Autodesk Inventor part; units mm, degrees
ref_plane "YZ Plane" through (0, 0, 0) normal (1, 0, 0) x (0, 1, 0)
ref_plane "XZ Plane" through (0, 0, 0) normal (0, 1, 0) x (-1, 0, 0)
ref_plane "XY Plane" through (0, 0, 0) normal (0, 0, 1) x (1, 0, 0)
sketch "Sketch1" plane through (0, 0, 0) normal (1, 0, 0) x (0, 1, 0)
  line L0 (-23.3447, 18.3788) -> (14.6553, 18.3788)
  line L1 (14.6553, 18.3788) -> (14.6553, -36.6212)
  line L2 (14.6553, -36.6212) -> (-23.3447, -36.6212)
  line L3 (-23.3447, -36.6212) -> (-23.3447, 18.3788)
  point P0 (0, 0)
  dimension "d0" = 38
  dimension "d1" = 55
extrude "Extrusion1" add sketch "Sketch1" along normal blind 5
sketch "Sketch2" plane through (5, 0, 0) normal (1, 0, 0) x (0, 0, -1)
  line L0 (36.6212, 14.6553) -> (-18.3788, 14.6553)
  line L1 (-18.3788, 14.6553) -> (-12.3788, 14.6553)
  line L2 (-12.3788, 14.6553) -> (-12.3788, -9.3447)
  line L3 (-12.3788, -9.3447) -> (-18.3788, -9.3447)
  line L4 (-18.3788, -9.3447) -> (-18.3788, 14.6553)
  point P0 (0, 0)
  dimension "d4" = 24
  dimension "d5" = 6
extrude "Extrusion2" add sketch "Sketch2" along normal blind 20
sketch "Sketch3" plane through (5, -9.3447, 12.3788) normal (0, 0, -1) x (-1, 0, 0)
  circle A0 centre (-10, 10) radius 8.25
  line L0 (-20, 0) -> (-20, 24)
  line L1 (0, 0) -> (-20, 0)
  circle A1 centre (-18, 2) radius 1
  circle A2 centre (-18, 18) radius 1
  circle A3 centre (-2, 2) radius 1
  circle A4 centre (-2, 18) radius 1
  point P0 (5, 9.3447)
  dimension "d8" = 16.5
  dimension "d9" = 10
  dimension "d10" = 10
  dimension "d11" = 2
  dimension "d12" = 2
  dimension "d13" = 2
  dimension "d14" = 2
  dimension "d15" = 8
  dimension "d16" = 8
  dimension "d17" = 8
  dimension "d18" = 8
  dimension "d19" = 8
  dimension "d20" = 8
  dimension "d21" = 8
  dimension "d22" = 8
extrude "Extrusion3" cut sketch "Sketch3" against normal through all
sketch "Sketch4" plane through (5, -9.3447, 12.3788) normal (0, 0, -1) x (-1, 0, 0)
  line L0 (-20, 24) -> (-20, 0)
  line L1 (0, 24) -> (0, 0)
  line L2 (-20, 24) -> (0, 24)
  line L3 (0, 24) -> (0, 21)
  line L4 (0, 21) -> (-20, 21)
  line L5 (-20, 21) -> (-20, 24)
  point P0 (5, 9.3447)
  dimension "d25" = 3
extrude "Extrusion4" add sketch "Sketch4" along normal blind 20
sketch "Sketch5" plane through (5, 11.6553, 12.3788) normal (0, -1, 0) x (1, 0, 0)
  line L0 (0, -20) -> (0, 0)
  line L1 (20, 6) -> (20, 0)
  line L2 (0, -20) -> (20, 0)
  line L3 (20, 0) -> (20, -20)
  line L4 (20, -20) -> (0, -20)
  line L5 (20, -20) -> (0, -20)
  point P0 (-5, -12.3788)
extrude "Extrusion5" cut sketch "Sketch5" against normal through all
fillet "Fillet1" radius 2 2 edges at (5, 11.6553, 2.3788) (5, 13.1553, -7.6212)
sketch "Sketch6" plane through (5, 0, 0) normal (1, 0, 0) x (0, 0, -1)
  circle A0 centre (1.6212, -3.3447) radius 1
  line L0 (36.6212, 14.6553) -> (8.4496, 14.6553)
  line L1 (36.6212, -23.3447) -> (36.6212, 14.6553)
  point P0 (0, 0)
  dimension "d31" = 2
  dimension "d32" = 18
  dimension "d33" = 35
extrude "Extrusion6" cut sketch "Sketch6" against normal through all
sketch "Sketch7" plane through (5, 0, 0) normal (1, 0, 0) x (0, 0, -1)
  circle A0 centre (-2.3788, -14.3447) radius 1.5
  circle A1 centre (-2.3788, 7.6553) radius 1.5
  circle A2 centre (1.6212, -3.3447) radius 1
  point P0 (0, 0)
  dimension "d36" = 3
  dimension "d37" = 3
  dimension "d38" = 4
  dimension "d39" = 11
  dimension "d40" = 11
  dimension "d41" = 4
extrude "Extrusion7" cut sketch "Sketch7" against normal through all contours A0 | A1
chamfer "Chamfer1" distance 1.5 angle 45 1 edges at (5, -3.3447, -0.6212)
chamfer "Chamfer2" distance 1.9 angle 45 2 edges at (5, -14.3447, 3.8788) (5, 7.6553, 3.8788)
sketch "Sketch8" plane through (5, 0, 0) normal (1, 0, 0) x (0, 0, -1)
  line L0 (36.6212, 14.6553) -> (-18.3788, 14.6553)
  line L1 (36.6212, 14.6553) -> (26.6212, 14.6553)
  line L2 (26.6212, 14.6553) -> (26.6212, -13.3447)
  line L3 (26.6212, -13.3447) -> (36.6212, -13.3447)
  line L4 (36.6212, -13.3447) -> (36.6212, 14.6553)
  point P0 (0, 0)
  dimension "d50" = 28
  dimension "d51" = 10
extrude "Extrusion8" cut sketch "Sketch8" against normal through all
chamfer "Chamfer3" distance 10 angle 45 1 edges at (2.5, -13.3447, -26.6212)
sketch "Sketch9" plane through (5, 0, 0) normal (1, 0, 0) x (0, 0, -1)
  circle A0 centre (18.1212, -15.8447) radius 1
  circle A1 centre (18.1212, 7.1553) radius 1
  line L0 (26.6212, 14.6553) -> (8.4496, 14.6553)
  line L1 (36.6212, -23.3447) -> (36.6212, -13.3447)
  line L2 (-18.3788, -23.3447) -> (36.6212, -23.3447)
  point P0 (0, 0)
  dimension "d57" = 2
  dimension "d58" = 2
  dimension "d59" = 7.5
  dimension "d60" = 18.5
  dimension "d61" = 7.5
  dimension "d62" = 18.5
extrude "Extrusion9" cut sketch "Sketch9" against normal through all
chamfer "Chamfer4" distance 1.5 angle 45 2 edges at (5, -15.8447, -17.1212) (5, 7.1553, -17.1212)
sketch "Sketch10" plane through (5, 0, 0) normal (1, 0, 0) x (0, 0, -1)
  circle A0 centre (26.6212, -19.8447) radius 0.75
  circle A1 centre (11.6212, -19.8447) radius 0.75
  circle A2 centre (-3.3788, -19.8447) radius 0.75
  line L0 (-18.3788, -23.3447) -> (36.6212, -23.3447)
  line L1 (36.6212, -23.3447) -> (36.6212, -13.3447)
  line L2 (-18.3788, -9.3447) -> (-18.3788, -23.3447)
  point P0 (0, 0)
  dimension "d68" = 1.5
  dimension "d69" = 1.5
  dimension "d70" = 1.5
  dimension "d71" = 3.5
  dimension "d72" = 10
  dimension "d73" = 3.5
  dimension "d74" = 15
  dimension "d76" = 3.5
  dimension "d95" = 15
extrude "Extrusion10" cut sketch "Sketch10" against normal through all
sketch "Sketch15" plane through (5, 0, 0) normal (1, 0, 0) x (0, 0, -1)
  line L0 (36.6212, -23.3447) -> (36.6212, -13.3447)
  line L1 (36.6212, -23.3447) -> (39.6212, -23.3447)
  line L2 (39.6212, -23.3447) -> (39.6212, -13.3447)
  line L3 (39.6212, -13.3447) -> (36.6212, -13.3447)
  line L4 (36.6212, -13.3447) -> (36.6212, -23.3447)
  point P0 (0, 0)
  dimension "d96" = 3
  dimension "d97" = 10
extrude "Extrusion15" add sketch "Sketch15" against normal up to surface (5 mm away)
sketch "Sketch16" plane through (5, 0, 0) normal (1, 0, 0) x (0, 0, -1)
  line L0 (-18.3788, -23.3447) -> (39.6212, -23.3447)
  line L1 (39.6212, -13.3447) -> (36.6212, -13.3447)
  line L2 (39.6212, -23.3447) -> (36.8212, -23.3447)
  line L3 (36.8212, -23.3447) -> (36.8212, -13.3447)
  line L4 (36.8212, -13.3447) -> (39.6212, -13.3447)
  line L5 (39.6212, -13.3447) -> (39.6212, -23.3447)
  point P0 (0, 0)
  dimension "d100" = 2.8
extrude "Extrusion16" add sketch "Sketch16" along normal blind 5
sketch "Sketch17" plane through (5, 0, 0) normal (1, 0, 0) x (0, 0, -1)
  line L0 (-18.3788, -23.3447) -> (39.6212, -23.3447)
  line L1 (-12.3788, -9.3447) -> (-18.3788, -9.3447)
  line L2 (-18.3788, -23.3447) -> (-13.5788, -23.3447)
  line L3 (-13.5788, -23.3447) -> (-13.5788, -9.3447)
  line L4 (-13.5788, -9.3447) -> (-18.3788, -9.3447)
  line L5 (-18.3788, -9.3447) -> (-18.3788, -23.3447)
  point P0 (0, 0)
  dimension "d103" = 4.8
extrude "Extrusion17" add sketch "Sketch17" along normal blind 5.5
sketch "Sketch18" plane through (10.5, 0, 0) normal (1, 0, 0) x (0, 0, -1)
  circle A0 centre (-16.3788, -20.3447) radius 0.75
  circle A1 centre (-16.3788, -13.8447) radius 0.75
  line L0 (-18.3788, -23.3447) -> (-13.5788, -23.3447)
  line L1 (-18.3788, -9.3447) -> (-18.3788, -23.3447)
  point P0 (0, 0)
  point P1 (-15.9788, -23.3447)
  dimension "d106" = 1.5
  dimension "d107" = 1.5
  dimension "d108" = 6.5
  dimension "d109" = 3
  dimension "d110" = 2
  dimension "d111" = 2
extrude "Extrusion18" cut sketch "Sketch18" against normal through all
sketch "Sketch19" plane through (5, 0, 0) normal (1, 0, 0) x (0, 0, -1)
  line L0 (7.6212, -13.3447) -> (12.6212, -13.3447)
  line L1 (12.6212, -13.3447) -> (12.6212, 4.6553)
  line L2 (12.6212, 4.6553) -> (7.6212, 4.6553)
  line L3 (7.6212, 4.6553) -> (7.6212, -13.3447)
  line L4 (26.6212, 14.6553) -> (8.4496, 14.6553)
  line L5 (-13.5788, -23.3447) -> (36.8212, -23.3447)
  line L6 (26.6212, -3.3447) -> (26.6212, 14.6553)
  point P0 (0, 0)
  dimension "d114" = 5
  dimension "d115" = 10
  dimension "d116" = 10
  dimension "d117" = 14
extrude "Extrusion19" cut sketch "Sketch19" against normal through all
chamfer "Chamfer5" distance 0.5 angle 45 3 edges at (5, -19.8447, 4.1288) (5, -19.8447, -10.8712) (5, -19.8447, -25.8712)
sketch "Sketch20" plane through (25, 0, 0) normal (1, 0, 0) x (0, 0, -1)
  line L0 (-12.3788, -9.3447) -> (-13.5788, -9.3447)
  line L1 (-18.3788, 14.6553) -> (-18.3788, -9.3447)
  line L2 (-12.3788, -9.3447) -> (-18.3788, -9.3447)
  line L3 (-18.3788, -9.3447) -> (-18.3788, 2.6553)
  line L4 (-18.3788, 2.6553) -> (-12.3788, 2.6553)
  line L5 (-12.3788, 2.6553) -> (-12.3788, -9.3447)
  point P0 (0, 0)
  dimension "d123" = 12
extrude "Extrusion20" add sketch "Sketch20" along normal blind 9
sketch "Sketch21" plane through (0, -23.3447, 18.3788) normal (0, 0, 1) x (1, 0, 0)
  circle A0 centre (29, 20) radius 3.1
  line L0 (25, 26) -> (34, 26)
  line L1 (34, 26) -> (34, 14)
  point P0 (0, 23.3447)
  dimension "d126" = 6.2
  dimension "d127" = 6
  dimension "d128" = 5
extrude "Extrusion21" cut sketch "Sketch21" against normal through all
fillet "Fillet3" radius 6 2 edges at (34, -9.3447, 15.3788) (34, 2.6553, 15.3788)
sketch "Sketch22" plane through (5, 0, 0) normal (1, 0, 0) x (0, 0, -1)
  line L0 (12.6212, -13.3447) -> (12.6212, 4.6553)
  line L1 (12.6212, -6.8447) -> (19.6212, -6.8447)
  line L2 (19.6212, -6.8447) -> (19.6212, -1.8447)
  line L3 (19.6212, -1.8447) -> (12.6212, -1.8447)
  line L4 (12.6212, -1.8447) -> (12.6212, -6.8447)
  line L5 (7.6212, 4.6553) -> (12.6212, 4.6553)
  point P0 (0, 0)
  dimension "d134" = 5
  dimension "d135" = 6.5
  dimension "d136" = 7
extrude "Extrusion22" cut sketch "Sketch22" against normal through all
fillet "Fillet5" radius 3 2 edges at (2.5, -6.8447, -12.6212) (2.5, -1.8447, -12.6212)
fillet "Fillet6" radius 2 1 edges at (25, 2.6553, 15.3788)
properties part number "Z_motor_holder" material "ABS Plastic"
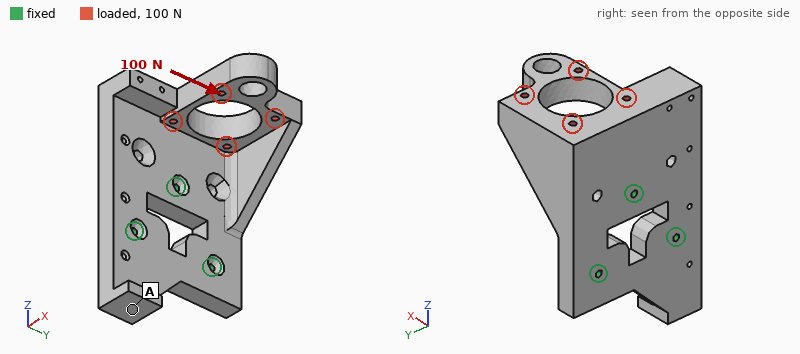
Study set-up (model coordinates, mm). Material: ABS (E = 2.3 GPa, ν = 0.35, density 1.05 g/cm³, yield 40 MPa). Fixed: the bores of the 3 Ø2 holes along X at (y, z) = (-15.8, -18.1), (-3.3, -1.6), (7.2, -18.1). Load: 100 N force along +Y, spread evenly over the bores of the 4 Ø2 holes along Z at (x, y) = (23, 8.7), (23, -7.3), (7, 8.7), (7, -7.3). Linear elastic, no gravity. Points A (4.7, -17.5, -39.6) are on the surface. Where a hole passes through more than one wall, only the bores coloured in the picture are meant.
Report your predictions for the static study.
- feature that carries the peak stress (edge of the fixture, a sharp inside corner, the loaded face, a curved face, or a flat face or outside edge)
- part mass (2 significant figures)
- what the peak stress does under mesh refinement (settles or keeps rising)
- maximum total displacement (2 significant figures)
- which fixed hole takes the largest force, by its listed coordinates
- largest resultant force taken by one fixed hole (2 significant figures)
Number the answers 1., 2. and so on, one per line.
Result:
1. edge of the fixture
2. 12 g
3. keeps rising
4. 0.83 mm
5. (-3.3, -1.6)
6. 110 N
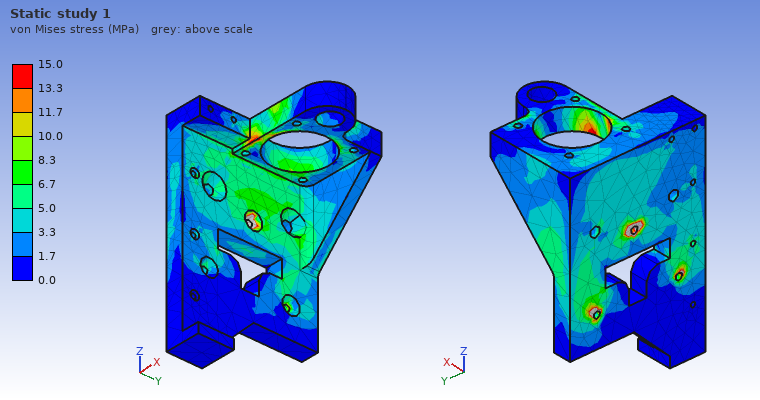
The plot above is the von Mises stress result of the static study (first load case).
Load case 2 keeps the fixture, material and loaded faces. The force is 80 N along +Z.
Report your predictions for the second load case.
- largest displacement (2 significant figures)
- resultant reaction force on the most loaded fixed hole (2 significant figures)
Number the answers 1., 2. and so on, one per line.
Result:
1. 0.84 mm
2. 54 N
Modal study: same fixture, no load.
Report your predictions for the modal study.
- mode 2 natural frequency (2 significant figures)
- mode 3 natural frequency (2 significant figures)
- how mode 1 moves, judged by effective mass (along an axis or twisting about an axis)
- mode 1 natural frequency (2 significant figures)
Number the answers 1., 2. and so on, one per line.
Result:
1. 1200 Hz
2. 2000 Hz
3. along X
4. 880 Hz
